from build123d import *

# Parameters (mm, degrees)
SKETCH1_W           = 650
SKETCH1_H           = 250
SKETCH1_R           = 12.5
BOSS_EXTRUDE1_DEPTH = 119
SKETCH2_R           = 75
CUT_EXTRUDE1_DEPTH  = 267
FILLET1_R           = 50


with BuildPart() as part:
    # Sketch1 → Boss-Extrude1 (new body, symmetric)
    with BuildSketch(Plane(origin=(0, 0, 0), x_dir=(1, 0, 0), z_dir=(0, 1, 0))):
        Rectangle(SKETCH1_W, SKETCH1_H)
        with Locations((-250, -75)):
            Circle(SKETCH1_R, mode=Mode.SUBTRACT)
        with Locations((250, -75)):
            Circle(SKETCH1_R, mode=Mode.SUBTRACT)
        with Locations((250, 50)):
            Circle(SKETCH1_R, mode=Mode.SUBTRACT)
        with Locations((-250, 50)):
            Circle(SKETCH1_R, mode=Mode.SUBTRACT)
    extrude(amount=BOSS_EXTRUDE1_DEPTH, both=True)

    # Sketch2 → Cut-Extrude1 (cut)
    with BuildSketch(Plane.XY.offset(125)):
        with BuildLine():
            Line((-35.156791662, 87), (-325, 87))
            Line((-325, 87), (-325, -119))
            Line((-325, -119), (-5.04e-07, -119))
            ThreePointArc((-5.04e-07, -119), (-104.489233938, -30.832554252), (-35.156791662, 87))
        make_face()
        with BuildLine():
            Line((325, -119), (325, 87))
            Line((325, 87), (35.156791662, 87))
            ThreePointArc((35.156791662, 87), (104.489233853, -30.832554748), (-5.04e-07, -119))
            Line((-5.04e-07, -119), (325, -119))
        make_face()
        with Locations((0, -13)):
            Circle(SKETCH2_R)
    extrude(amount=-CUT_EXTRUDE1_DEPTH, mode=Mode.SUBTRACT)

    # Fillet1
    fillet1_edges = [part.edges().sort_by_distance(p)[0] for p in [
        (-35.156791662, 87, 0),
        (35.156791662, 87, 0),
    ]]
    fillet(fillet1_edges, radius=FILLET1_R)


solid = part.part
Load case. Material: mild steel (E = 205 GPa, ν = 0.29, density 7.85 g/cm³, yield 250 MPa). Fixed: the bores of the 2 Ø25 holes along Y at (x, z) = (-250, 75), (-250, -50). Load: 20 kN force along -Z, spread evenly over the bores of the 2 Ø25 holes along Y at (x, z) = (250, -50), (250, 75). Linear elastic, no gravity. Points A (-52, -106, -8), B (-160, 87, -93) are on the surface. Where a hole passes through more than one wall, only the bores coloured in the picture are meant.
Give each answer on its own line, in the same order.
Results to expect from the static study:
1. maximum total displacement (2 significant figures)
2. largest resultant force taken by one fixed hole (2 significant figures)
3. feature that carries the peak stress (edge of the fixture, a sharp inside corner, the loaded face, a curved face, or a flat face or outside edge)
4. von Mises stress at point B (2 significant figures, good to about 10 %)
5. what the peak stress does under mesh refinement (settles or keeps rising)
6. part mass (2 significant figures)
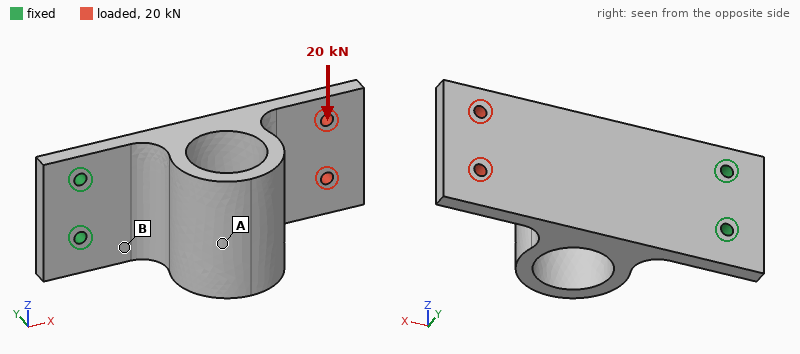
0.16 mm
73 kN
edge of the fixture
21 MPa
keeps rising
82 kg
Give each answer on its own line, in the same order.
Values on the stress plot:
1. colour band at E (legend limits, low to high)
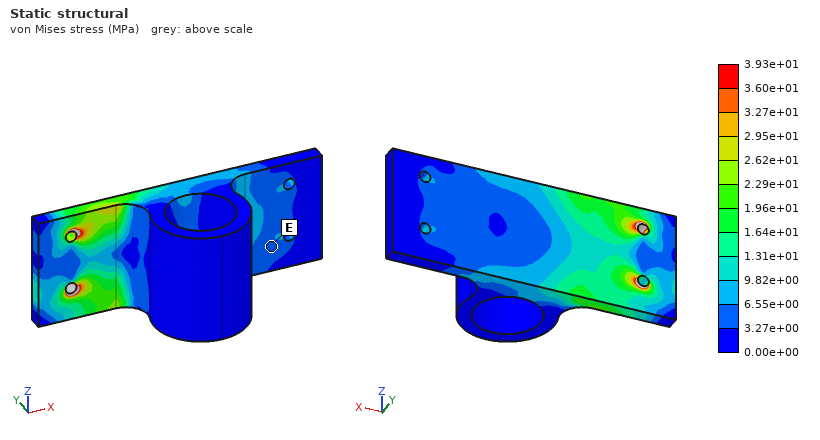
3.27e+00 to 6.55e+00 MPa
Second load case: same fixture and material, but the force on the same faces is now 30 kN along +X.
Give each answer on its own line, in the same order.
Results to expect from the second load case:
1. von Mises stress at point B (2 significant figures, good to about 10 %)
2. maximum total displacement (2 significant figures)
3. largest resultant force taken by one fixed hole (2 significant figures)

2.6 MPa
34 µm
15 kN
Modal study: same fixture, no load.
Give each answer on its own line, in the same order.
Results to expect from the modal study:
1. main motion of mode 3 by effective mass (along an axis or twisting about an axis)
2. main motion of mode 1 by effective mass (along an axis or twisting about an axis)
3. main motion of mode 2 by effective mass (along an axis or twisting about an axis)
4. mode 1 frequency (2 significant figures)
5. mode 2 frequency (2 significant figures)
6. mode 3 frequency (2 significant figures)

along Z
along Y
along Z
72 Hz
280 Hz
440 Hz
